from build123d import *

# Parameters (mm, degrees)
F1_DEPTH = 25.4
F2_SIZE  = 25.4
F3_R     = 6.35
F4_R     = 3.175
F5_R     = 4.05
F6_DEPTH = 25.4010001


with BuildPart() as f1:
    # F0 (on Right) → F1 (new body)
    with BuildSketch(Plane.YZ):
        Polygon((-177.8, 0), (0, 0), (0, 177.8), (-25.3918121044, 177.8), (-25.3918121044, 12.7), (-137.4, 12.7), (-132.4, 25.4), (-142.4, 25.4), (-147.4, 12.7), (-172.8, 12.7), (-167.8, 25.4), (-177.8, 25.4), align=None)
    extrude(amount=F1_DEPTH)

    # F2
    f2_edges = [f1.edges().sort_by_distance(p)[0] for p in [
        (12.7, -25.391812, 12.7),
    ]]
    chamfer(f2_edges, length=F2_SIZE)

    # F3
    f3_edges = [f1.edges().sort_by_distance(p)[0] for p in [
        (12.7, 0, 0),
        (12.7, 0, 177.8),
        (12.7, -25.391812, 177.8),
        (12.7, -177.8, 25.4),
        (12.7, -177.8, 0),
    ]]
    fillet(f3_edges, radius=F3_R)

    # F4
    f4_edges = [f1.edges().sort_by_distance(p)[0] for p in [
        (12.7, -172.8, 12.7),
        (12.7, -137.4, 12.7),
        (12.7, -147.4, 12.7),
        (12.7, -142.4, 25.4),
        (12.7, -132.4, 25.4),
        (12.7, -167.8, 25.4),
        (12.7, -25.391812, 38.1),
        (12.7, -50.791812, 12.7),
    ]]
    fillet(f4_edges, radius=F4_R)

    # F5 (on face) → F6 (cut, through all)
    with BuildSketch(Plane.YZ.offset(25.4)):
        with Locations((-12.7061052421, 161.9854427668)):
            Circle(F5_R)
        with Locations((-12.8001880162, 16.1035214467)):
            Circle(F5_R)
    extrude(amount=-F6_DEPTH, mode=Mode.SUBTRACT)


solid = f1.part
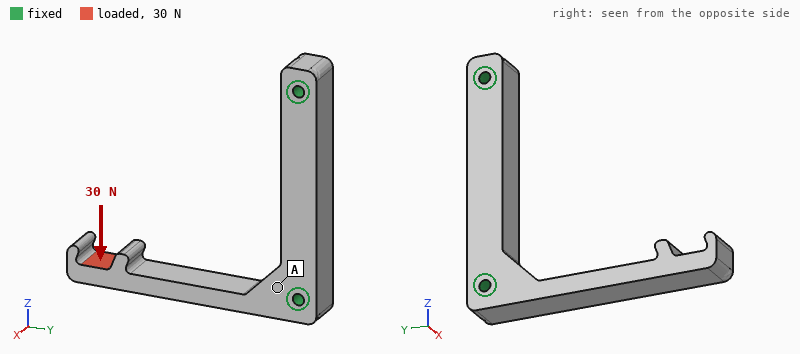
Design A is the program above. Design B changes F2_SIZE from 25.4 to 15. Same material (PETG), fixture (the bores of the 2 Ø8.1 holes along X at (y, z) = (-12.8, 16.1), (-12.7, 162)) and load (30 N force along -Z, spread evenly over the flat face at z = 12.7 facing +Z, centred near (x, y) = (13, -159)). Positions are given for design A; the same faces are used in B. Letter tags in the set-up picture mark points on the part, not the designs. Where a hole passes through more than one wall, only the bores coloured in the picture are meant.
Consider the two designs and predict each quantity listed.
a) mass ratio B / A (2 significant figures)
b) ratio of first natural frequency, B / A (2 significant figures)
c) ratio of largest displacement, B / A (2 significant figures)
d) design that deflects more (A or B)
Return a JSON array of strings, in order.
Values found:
["0.97", "0.88", "1.2", "B"]
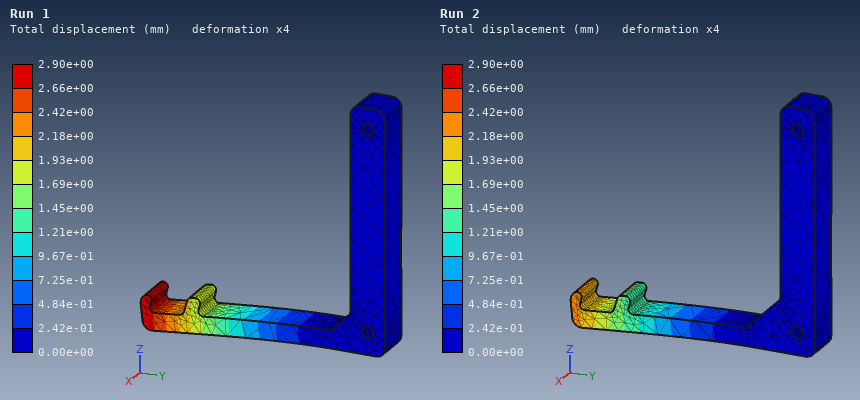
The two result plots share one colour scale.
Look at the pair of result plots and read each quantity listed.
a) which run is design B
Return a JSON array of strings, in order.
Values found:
["Run 1"]
